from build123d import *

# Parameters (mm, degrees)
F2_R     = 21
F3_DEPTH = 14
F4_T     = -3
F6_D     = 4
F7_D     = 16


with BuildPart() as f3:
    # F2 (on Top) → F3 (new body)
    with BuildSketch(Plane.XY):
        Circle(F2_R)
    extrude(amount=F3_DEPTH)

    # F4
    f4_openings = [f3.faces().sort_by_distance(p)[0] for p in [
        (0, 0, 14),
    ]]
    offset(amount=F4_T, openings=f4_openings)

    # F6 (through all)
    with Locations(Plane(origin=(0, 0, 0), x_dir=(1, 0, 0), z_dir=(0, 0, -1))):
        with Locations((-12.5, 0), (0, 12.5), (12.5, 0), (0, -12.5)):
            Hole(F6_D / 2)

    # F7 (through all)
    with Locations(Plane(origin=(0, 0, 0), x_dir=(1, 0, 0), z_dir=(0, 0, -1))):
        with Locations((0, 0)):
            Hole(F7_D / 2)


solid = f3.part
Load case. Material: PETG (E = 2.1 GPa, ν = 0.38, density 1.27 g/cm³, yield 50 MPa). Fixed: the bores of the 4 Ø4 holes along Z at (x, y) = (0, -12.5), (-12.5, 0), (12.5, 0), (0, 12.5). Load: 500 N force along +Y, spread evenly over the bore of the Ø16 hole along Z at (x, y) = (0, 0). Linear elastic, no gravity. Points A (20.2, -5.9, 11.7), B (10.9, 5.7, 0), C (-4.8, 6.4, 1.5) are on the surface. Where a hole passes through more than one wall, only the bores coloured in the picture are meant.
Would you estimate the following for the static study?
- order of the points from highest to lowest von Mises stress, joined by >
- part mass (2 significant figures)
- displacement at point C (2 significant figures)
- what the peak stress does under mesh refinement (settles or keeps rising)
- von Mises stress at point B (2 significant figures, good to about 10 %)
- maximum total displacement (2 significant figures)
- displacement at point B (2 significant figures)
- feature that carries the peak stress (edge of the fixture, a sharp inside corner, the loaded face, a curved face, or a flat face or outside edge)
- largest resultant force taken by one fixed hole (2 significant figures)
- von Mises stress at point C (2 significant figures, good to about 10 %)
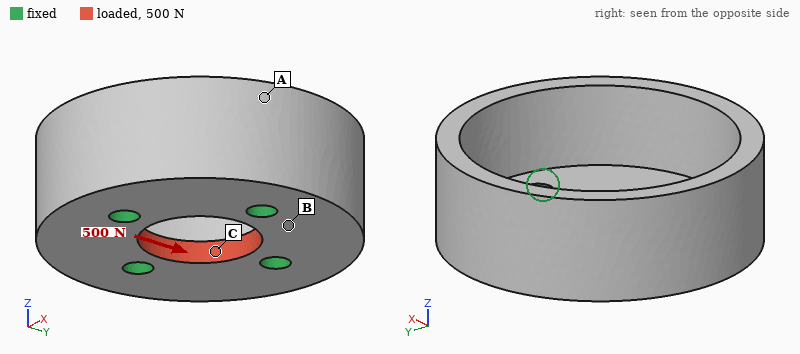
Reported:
C > B > A
9.5 g
15 µm
keeps rising
2.0 MPa
17 µm
7.0 µm
edge of the fixture
130 N
4.4 MPa
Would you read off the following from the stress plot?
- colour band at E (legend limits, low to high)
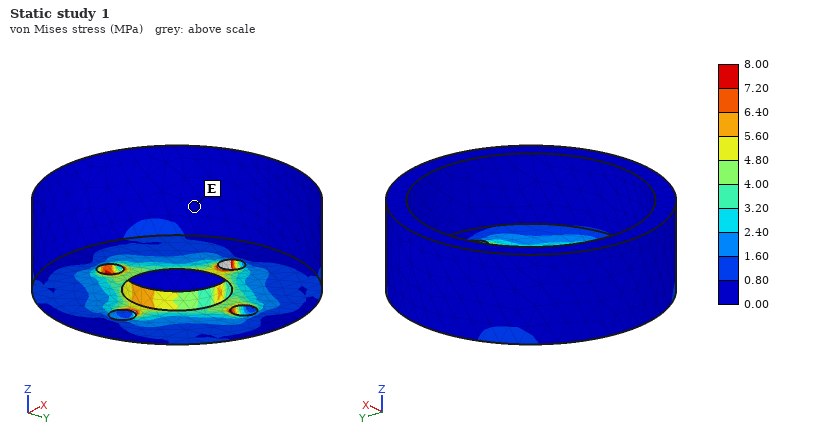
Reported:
0.00 to 0.80 MPa
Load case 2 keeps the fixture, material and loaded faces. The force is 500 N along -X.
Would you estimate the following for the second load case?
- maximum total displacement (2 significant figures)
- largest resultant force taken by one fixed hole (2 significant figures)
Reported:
17 µm
130 N
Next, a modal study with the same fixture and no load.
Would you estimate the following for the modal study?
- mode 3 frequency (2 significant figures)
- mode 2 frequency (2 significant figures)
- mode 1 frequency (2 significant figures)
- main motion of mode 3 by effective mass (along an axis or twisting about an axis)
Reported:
3500 Hz
3300 Hz
2500 Hz
along Y
